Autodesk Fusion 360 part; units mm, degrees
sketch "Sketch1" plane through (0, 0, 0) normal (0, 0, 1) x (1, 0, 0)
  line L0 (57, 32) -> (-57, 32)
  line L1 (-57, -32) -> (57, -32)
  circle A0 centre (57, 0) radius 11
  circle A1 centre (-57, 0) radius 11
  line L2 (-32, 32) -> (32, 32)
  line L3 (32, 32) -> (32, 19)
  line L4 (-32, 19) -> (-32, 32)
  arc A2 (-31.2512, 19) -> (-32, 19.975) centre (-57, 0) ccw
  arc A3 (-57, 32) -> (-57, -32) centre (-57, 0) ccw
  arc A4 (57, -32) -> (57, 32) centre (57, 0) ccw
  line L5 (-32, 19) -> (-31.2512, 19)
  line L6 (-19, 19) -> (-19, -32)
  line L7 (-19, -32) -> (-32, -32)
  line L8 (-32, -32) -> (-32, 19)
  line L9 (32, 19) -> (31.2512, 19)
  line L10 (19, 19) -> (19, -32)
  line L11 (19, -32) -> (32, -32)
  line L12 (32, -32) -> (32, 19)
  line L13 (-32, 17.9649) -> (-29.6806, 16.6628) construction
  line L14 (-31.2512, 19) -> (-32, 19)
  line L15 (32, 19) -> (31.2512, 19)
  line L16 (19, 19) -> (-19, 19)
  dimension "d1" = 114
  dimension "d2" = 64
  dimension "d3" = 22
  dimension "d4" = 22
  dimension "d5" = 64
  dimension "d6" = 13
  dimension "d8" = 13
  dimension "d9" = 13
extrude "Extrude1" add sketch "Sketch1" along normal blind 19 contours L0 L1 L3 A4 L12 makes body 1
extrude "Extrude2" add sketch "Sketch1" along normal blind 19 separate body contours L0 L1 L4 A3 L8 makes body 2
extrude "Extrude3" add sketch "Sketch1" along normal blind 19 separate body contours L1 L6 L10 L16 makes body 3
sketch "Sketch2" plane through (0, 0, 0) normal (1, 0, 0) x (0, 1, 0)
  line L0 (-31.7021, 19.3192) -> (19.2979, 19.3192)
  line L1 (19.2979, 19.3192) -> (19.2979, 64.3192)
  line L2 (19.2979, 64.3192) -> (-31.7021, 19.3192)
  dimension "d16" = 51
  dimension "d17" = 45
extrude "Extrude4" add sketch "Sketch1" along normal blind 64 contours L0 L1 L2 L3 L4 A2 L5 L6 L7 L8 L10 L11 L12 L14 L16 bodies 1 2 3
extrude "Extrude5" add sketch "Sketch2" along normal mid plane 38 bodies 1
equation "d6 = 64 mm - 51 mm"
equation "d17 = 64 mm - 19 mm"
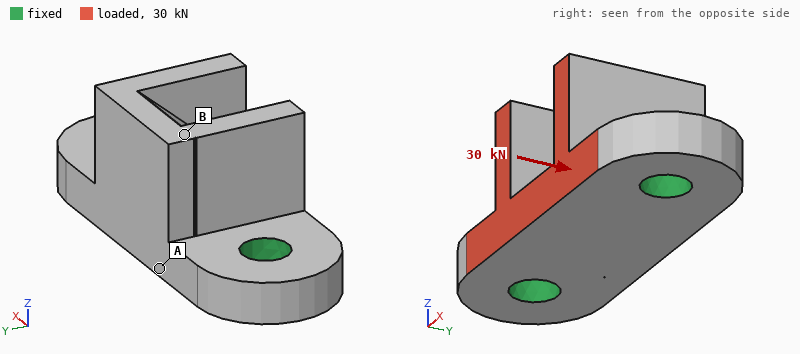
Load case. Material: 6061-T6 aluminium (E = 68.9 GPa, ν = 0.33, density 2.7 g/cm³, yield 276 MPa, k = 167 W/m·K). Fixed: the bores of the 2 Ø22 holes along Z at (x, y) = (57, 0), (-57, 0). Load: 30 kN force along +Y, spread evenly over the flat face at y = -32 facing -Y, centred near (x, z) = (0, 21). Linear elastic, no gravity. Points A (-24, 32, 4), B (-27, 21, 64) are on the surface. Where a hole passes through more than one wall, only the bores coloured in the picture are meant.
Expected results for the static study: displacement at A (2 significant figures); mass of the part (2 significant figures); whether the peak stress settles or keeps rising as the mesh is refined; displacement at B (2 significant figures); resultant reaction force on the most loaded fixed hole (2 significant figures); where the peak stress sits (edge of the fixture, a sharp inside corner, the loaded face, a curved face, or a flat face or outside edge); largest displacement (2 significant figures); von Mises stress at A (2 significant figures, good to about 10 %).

32 µm
880 g
keeps rising
79 µm
15 kN
edge of the fixture
89 µm
21 MPa
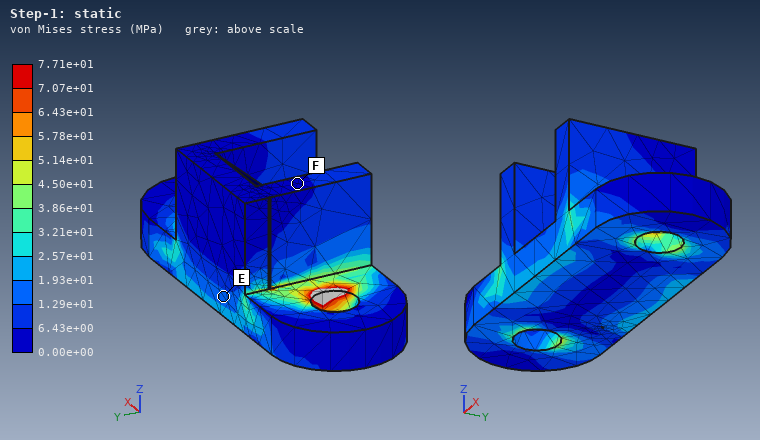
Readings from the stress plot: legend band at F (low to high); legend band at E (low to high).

0.00e+00 to 6.43e+00 MPa
1.29e+01 to 1.93e+01 MPa
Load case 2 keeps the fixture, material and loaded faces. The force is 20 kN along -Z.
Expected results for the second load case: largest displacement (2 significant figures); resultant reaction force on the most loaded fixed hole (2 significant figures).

0.12 mm
10 kN
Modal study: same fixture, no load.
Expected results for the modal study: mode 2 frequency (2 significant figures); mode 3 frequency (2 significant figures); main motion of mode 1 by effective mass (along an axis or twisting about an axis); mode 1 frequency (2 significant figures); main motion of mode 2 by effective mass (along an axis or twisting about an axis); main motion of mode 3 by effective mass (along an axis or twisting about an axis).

6300 Hz
7000 Hz
along Y
3500 Hz
along Z
along X
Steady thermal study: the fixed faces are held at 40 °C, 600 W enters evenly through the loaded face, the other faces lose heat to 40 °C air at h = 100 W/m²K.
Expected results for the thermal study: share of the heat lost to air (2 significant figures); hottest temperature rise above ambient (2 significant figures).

16 %
61 K
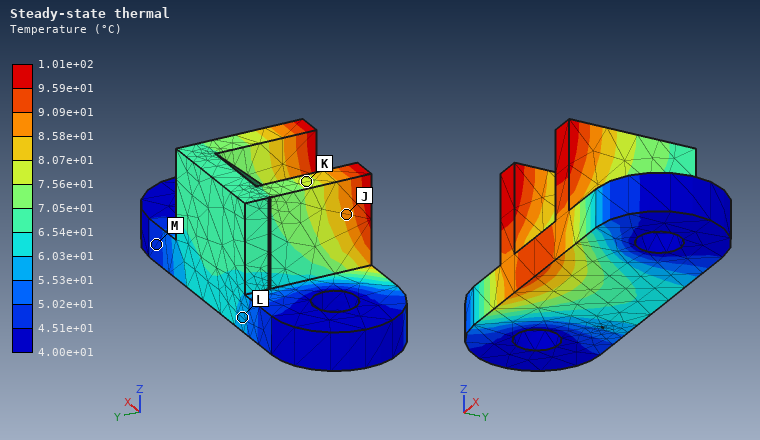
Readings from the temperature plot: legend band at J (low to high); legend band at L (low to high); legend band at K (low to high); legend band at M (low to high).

8.58e+01 to 9.09e+01 °C
5.53e+01 to 6.03e+01 °C
7.56e+01 to 8.07e+01 °C
4.51e+01 to 5.02e+01 °C
